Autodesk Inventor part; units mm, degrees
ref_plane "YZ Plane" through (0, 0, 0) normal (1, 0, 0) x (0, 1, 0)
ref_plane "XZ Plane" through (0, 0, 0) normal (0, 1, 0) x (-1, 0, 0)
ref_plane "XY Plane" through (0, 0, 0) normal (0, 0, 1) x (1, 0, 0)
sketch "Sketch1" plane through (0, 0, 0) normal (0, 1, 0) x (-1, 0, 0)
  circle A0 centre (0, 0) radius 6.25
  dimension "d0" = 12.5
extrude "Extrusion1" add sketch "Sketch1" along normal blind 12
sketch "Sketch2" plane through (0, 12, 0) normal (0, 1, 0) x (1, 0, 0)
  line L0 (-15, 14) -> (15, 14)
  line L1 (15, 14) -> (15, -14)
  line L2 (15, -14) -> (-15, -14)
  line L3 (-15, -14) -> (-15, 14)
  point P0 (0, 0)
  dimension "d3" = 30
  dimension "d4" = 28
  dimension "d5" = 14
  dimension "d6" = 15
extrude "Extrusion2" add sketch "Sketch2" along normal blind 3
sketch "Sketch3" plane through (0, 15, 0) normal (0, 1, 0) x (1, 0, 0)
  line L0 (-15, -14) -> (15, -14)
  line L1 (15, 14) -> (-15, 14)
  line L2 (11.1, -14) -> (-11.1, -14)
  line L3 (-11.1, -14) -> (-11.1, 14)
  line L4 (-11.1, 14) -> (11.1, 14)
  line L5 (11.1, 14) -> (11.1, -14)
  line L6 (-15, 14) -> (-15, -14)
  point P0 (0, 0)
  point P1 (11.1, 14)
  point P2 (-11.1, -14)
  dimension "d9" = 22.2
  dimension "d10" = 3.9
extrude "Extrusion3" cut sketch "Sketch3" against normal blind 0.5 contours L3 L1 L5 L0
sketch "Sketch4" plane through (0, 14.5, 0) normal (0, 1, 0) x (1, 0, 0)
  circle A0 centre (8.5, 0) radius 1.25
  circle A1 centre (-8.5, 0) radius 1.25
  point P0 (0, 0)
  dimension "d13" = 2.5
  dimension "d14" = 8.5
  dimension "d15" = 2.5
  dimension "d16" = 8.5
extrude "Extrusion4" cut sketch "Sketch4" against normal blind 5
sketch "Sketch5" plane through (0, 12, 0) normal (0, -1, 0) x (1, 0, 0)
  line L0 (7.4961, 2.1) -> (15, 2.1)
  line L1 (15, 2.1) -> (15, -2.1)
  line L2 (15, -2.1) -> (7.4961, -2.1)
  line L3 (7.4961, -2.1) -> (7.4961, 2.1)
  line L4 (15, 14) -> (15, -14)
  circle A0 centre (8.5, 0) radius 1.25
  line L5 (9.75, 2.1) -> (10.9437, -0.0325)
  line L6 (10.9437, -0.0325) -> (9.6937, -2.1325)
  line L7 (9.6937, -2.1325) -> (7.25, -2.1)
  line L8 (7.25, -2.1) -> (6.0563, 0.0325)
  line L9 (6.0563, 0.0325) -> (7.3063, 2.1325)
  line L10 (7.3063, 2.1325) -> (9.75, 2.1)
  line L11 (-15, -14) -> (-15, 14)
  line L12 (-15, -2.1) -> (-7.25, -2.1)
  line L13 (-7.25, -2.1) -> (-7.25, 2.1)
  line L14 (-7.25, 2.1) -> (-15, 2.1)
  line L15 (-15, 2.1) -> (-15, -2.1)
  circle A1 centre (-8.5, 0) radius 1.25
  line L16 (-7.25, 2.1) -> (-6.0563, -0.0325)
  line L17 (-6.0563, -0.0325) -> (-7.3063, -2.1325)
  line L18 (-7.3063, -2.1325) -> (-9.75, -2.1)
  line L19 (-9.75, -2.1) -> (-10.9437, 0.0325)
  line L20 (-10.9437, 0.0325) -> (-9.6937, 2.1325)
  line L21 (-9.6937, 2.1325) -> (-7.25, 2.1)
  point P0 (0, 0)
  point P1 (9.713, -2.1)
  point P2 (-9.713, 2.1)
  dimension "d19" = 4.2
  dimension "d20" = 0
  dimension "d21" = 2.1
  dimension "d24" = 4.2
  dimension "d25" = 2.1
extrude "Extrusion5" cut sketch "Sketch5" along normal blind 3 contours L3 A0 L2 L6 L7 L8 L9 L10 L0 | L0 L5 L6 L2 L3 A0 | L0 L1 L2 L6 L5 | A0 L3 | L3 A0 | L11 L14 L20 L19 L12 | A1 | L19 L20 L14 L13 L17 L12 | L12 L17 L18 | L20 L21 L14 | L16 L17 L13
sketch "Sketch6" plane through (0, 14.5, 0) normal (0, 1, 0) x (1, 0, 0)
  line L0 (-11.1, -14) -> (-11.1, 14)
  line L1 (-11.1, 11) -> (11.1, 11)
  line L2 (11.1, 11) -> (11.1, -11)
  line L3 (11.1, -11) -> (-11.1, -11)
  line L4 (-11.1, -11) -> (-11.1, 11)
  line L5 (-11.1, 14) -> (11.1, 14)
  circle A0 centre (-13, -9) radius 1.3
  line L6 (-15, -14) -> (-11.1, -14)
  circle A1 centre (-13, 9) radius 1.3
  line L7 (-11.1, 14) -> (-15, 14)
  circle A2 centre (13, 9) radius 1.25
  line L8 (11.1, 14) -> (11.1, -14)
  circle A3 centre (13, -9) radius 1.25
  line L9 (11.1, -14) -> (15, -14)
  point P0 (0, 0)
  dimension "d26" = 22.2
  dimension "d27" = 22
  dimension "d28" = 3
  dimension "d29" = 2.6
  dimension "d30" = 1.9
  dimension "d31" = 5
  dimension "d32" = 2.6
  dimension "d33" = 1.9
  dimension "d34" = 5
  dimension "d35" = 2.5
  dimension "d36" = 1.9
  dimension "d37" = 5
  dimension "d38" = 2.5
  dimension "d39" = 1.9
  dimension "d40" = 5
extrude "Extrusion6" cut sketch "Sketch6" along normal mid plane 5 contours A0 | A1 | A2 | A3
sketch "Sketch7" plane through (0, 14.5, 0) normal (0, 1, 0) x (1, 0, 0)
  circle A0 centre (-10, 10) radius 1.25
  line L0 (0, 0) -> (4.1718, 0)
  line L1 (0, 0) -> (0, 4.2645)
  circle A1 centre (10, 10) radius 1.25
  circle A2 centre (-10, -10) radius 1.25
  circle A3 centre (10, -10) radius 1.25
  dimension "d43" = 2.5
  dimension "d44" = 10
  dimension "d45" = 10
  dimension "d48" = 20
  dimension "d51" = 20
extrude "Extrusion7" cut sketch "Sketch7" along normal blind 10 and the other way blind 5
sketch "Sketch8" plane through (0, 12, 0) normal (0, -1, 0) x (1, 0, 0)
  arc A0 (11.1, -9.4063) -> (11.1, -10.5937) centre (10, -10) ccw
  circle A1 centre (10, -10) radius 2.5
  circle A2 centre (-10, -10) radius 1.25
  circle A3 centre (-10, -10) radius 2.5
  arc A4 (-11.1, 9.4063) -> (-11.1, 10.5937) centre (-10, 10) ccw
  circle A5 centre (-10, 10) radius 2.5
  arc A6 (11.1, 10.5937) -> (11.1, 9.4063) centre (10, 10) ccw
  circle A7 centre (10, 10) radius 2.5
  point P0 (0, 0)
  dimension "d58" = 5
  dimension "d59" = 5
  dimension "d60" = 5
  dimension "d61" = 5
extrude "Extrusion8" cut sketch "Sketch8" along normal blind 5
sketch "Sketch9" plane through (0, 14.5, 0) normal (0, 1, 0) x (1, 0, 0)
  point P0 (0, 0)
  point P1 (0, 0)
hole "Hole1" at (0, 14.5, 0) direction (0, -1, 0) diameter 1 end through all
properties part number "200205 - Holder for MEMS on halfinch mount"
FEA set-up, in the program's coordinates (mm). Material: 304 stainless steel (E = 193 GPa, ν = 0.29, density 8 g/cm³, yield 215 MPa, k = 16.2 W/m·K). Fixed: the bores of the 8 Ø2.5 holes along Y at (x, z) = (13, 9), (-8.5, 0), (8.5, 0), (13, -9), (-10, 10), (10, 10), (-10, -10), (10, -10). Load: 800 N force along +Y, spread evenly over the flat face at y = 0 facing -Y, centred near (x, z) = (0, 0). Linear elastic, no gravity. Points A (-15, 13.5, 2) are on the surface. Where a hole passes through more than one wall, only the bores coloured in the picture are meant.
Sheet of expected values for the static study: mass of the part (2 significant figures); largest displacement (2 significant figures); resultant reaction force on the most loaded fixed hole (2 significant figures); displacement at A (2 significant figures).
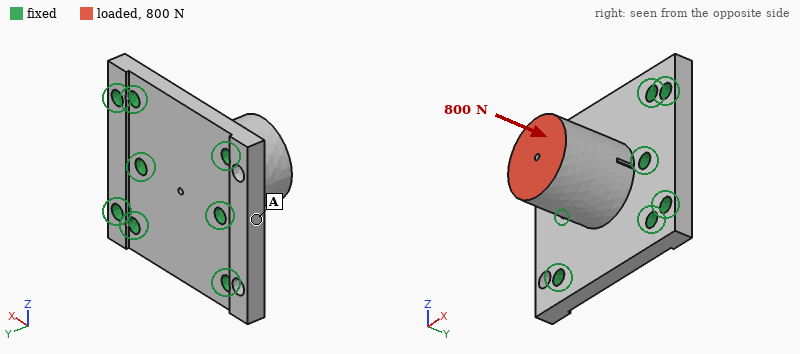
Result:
28 g
1.7 µm
350 N
0.32 µm
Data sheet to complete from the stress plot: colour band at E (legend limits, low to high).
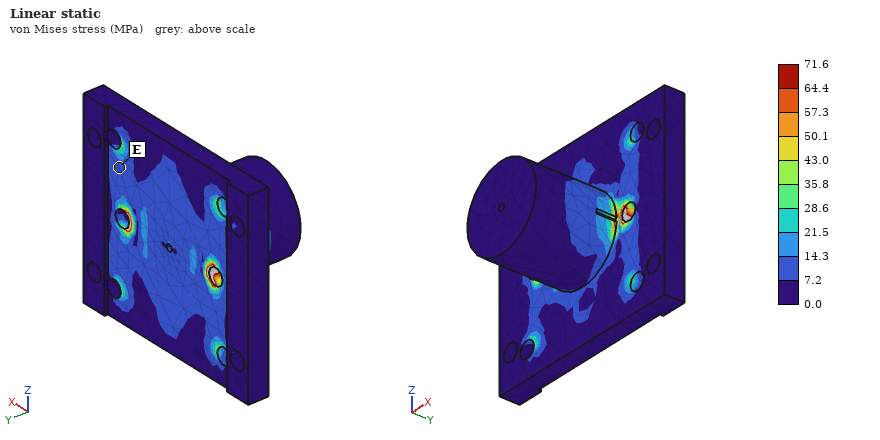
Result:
7.2 to 14.3 MPa
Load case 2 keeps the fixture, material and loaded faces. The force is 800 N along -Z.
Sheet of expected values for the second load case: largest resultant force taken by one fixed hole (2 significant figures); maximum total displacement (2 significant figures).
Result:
290 N
19 µm
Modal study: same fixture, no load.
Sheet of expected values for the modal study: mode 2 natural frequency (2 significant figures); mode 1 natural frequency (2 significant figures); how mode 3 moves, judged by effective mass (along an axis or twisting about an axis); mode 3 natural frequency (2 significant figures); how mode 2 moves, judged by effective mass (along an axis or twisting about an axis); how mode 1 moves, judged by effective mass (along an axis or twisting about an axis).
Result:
24 kHz
15 kHz
along Y
29 kHz
along X
along Z
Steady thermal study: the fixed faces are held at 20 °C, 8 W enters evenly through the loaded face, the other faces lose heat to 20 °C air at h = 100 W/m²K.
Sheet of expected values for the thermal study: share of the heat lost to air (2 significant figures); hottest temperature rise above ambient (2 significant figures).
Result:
35 %
61 K
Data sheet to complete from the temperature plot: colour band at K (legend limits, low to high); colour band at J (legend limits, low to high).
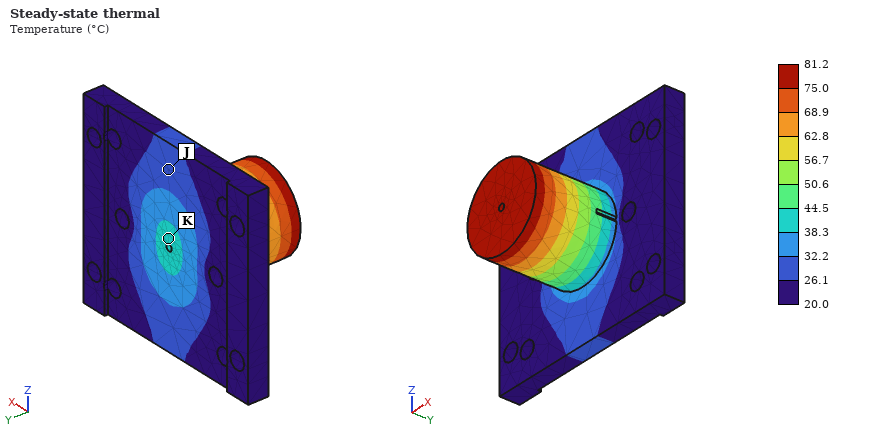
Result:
38.3 to 44.5 °C
26.1 to 32.2 °C
